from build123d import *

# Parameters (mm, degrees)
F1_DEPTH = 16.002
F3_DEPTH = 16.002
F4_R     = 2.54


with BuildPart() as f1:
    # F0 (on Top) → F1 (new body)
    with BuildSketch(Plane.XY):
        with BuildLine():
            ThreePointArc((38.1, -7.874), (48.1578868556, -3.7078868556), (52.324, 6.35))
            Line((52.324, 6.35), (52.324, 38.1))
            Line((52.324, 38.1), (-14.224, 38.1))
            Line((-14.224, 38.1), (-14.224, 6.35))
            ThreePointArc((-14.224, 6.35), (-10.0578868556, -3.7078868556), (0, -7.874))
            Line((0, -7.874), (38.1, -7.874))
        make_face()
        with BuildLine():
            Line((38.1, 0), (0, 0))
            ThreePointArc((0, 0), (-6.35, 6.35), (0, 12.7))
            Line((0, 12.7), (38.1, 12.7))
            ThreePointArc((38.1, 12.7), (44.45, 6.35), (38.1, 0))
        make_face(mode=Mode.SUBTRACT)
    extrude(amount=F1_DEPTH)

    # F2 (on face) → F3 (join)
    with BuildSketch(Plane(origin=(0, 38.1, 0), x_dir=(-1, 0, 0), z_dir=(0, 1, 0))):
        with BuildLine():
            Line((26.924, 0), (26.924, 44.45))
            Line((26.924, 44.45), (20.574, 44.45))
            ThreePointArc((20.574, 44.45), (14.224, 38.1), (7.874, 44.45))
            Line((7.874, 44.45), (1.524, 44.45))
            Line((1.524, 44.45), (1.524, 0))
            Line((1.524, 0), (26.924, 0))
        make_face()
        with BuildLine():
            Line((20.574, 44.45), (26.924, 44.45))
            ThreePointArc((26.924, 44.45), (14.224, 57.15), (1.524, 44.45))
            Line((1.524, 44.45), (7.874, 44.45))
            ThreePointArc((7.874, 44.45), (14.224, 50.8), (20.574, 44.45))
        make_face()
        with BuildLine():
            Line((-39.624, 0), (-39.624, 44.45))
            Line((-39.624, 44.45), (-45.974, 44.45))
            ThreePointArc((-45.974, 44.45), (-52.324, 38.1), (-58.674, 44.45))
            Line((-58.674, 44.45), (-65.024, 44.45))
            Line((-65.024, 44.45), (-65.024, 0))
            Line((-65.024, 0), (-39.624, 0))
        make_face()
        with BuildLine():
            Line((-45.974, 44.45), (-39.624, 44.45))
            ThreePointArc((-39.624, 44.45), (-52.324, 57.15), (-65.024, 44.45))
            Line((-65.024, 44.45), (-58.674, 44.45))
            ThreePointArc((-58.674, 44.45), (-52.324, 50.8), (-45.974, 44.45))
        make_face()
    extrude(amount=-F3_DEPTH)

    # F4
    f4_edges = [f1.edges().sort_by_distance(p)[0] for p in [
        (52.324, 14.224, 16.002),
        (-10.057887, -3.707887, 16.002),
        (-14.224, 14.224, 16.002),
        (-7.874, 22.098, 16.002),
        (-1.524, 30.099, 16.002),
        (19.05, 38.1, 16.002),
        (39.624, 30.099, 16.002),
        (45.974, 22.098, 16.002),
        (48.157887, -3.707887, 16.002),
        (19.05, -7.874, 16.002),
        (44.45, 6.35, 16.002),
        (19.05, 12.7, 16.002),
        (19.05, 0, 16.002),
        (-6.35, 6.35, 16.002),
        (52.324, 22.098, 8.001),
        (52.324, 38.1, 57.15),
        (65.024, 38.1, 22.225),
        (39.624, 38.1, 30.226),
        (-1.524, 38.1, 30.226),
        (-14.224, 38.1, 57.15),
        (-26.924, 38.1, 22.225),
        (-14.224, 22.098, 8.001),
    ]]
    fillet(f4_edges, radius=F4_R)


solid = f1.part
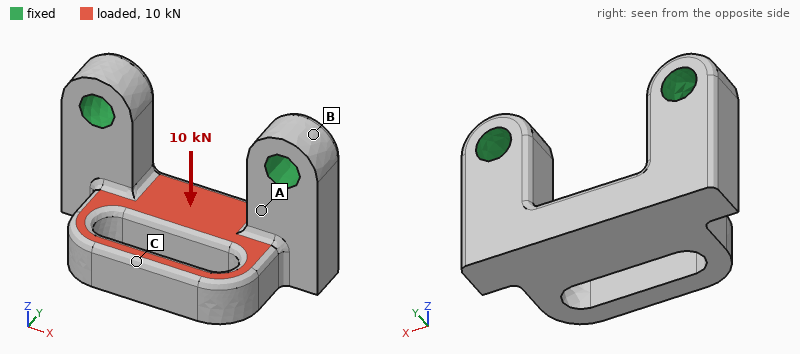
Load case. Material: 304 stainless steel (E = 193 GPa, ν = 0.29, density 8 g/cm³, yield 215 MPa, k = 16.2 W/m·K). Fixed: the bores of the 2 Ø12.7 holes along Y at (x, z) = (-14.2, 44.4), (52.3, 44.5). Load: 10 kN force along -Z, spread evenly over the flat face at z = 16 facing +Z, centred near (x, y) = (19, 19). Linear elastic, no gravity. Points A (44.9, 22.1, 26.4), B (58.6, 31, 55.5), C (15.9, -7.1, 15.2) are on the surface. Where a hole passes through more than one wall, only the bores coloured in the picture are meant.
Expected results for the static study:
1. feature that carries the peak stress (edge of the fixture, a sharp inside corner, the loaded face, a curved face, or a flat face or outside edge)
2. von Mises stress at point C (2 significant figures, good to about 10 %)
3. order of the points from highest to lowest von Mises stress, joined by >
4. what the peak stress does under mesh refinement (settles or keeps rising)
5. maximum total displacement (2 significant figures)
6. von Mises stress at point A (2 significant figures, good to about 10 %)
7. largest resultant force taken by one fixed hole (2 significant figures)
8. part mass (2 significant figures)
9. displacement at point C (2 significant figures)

a sharp inside corner
26 MPa
A > C > B
keeps rising
71 µm
79 MPa
5.4 kN
570 g
63 µm
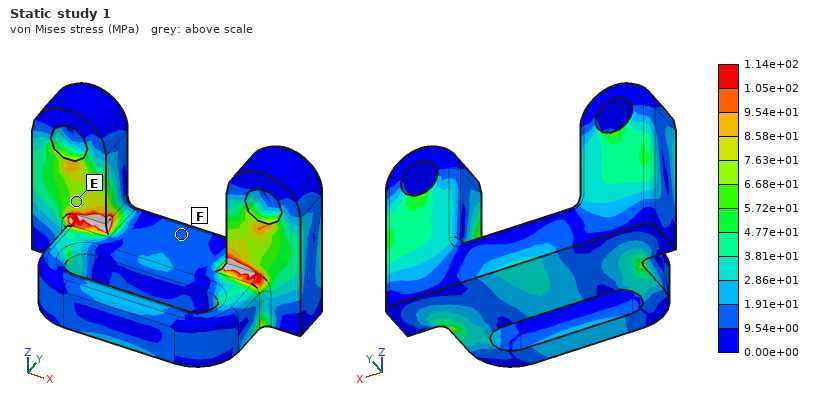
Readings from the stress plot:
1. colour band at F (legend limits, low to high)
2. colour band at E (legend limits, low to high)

9.54e+00 to 1.91e+01 MPa
6.68e+01 to 7.63e+01 MPa
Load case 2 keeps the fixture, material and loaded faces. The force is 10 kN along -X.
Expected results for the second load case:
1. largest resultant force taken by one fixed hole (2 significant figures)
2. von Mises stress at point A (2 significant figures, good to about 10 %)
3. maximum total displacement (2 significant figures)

5.3 kN
40 MPa
36 µm
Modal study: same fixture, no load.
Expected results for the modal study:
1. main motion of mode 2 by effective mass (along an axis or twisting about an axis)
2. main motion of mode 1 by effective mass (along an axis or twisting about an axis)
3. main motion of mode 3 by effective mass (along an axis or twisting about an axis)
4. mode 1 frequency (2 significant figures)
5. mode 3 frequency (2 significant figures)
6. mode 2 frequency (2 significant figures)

along X
along Y
along Y
3100 Hz
6800 Hz
5300 Hz
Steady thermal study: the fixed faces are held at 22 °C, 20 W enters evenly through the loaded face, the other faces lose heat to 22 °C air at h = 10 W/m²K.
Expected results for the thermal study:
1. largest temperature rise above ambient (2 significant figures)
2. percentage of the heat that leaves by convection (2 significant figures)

60 K
24 %
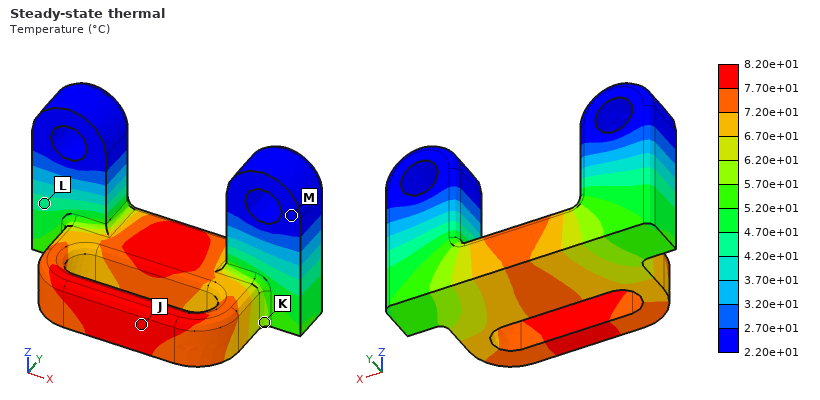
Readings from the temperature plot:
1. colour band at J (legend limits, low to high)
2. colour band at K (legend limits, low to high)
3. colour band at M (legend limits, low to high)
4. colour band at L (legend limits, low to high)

7.70e+01 to 8.20e+01 °C
5.70e+01 to 6.20e+01 °C
2.20e+01 to 2.70e+01 °C
4.20e+01 to 4.70e+01 °C
